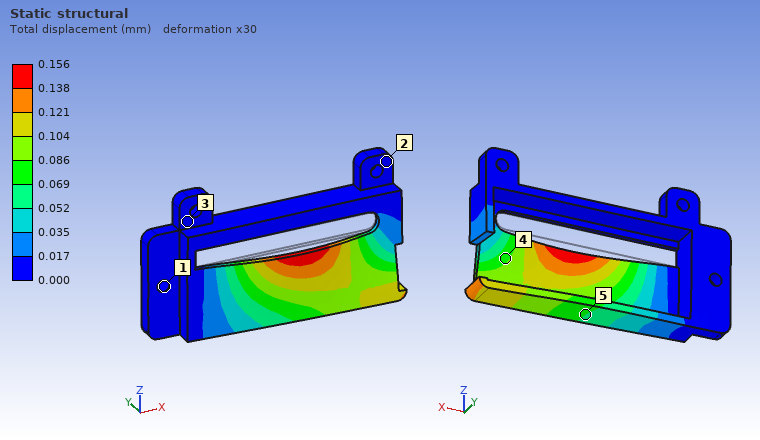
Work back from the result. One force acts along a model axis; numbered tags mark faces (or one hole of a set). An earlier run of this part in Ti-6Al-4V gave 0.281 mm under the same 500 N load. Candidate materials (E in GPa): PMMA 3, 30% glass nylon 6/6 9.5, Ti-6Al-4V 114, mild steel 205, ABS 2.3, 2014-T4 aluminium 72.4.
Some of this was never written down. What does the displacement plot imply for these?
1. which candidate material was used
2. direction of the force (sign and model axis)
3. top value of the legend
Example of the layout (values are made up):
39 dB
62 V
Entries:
mild steel
-Y
0.156 mm
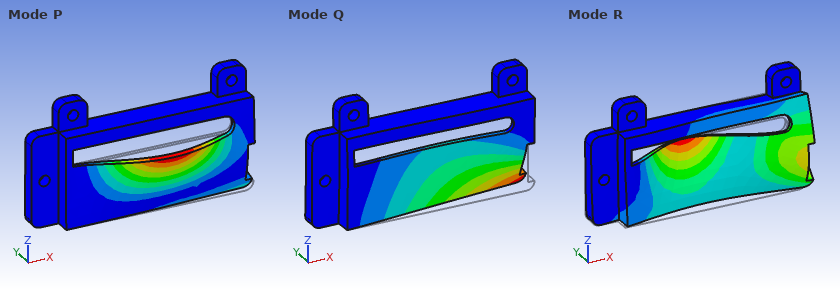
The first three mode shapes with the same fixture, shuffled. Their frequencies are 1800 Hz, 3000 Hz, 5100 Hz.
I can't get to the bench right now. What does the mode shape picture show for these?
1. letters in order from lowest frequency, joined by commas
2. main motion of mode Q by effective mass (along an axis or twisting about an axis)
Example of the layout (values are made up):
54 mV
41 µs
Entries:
Q, P, R
along Y
